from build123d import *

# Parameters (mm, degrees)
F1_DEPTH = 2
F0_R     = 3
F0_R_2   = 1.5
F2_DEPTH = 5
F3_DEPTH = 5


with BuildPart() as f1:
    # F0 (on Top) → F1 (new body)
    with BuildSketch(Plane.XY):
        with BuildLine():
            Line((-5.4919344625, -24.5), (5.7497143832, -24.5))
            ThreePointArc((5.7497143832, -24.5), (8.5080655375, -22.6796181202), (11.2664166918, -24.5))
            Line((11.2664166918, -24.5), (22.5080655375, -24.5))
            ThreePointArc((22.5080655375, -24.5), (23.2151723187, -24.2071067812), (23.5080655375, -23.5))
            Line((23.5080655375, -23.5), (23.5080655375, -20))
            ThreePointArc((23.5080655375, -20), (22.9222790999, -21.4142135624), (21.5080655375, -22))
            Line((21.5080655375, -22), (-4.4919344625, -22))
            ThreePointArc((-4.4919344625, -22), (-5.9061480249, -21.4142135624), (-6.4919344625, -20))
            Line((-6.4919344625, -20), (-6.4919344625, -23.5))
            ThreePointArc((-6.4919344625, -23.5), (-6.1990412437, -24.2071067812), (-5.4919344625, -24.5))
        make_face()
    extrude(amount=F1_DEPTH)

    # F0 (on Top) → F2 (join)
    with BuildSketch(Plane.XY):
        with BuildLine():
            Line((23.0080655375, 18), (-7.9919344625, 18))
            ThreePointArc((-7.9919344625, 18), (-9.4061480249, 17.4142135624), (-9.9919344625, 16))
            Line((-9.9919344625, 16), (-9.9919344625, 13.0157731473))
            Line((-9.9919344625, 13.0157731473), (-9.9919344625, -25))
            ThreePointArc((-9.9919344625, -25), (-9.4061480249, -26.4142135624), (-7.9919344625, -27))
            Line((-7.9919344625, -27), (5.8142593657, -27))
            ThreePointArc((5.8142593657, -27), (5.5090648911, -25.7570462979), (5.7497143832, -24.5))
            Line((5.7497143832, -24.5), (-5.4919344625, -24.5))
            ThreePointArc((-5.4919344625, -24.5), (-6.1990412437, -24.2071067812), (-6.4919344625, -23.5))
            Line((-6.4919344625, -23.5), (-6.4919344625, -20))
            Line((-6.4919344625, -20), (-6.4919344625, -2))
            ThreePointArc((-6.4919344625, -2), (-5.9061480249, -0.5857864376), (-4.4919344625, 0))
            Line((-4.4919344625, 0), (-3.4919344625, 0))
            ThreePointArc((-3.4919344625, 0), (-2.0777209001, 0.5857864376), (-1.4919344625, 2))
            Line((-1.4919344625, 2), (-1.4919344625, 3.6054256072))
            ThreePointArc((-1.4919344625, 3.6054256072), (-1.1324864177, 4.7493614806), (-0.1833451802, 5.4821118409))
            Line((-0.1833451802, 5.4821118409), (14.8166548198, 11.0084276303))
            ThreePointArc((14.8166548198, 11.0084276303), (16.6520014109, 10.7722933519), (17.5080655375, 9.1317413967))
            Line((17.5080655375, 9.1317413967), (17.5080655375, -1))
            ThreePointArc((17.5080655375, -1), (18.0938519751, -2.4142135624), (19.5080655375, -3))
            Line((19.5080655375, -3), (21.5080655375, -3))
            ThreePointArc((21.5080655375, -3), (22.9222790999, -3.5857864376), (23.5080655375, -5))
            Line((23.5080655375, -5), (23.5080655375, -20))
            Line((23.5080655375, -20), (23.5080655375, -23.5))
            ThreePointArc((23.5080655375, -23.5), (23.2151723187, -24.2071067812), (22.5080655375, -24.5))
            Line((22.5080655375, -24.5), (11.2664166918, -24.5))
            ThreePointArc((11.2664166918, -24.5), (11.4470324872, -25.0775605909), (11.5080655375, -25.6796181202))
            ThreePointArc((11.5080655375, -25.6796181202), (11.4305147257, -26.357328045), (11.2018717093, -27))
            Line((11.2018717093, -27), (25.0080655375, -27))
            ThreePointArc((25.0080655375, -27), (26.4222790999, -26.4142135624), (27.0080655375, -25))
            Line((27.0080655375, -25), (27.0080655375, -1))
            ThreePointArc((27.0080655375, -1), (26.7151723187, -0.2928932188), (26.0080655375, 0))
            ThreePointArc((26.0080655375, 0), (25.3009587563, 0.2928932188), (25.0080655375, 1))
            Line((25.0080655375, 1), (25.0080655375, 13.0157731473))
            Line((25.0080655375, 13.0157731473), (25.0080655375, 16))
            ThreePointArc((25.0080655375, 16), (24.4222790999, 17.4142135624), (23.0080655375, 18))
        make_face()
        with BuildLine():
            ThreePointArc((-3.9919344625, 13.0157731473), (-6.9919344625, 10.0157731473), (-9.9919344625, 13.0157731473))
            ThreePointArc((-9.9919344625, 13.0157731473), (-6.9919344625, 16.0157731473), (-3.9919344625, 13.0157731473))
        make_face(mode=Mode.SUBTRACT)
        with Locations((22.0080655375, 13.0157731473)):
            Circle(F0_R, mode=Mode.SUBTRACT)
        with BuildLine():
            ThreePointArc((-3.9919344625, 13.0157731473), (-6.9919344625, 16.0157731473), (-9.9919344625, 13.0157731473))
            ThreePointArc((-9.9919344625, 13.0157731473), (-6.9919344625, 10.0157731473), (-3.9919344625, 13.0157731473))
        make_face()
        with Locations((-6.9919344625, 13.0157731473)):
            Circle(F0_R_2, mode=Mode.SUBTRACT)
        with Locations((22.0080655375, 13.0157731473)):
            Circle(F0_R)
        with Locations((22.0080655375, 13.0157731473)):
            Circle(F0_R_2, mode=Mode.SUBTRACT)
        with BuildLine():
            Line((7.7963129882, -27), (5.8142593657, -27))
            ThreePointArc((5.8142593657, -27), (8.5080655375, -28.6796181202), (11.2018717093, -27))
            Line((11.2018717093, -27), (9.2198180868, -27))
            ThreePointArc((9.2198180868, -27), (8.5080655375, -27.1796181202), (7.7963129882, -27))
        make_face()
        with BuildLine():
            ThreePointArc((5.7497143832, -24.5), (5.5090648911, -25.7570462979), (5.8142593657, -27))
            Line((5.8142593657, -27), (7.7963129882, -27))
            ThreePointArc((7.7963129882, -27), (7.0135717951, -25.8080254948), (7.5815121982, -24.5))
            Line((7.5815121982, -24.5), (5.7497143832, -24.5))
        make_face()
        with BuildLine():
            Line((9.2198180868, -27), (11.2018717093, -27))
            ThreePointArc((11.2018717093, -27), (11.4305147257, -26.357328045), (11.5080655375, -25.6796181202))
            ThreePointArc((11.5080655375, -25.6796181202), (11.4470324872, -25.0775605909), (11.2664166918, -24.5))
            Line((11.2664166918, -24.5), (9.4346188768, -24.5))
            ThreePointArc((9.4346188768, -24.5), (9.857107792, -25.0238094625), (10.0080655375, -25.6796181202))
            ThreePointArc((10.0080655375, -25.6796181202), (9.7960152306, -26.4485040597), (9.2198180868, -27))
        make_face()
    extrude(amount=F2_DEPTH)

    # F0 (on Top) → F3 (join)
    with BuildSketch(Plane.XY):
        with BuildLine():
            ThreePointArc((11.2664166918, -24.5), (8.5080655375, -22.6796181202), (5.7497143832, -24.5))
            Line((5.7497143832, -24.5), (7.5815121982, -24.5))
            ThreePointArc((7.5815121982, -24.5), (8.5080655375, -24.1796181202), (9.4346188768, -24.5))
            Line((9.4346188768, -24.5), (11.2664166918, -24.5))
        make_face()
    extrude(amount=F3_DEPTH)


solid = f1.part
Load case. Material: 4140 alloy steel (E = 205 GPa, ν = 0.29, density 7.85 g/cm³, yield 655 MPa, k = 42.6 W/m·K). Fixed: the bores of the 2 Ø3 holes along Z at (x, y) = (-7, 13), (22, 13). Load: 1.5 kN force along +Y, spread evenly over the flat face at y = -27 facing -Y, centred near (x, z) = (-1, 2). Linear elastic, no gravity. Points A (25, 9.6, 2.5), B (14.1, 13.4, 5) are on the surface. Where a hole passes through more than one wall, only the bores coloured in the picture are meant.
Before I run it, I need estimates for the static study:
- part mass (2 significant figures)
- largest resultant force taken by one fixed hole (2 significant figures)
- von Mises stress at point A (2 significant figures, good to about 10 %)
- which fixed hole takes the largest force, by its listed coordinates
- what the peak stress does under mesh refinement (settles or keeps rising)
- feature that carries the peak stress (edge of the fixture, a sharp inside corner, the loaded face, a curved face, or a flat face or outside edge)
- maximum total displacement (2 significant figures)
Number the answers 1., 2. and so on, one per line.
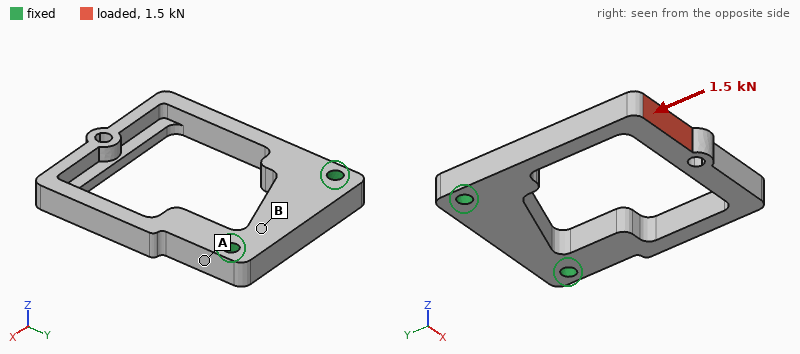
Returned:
1. 30 g
2. 1.2 kN
3. 75 MPa
4. (-7, 13)
5. keeps rising
6. a sharp inside corner
7. 87 µm
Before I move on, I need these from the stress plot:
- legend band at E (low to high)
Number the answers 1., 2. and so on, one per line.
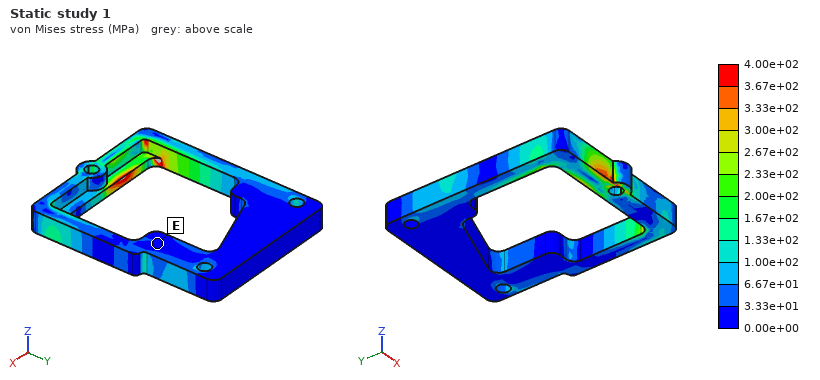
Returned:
1. 0.00e+00 to 3.33e+01 MPa
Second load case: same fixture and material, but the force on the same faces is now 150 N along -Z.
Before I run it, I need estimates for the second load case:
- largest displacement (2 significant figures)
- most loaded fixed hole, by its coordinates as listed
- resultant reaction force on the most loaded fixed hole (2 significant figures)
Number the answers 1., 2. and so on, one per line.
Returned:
1. 0.17 mm
2. (-7, 13)
3. 120 N
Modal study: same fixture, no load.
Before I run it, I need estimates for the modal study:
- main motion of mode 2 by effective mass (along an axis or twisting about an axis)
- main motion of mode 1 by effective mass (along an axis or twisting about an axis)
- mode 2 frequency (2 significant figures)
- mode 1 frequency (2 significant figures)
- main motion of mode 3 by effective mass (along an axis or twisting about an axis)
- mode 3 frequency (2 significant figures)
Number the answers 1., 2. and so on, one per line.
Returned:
1. along X
2. along Z
3. 3400 Hz
4. 2200 Hz
5. twisting about Y
6. 4100 Hz
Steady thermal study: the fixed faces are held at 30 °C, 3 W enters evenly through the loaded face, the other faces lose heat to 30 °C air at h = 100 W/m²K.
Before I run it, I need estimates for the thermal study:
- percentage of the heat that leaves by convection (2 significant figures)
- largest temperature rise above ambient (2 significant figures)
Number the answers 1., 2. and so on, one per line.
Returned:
1. 79 %
2. 35 K
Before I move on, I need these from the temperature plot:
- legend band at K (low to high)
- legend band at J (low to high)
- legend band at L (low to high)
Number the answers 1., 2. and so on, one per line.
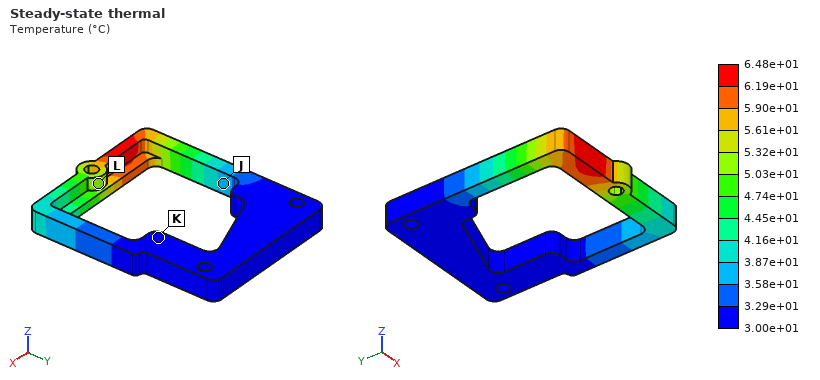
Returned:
1. 3.00e+01 to 3.29e+01 °C
2. 3.58e+01 to 3.87e+01 °C
3. 5.03e+01 to 5.32e+01 °C
